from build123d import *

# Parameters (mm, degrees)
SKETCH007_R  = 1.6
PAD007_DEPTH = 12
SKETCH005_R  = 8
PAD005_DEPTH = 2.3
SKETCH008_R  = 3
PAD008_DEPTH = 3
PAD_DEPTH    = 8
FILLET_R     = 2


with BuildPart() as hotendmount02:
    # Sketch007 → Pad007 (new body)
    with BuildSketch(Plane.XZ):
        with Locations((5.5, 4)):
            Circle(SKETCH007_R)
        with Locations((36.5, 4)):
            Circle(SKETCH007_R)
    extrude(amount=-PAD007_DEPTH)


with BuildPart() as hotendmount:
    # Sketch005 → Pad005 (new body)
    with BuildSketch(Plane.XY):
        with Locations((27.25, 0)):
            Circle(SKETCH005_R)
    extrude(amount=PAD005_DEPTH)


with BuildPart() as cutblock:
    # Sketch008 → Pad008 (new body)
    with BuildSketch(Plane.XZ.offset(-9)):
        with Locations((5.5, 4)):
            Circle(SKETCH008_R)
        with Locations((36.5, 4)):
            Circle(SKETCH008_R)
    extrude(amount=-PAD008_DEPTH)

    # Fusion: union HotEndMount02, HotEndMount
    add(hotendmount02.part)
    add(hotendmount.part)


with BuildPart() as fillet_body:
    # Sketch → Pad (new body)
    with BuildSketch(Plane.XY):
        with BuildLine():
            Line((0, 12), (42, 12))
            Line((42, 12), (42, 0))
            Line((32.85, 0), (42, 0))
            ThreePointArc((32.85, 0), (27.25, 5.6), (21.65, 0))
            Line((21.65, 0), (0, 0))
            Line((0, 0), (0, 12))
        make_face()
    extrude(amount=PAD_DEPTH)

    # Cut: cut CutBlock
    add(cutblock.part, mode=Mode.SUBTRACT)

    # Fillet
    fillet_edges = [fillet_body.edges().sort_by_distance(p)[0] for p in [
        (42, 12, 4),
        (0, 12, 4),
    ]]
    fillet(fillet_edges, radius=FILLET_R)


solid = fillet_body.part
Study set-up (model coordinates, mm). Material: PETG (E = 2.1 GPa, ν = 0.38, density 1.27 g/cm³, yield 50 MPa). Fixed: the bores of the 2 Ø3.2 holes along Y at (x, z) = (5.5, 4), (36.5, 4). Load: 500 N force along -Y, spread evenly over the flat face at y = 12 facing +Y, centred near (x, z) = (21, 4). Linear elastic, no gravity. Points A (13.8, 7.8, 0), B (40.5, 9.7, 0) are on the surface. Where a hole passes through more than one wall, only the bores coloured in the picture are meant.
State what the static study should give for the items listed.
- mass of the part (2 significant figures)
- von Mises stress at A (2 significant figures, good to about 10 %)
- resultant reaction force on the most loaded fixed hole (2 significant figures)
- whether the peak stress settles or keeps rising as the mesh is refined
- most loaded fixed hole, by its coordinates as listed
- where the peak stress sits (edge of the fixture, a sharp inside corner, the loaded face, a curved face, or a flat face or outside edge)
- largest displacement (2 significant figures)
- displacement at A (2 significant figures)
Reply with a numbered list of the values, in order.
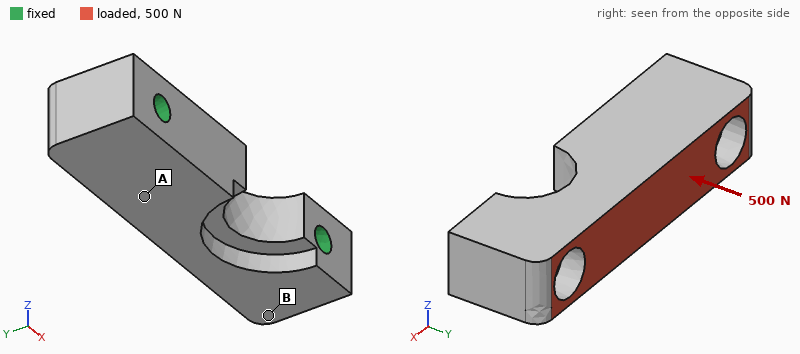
1. 4.1 g
2. 4.2 MPa
3. 290 N
4. keeps rising
5. (5.5, 4)
6. edge of the fixture
7. 83 µm
8. 49 µm
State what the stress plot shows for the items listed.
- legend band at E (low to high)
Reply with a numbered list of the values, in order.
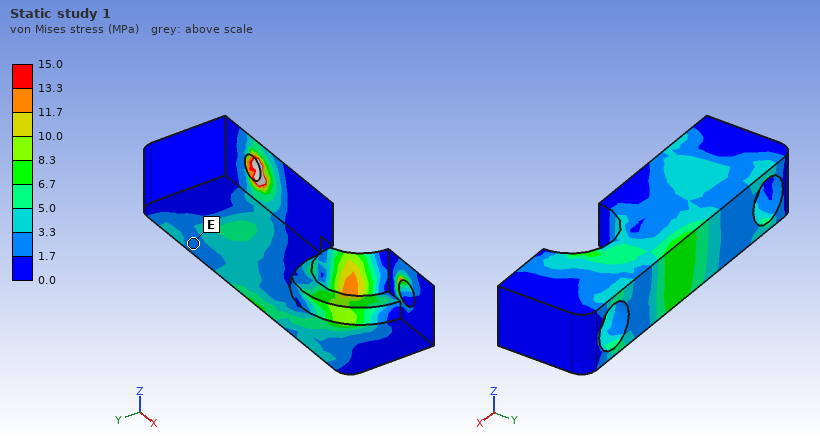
1. 1.7 to 3.3 MPa
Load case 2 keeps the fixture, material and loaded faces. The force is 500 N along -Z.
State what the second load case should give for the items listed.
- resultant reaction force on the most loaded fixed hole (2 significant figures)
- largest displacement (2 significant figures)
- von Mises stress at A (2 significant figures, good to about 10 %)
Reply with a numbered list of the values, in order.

1. 250 N
2. 0.26 mm
3. 8.8 MPa
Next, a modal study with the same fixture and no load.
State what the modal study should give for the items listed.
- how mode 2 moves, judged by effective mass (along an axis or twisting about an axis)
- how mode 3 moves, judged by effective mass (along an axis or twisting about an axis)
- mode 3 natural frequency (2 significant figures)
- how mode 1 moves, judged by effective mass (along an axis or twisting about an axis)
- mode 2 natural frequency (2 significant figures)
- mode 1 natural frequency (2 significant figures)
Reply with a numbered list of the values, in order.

1. along Y
2. twisting about X
3. 9800 Hz
4. along Z
5. 8400 Hz
6. 6500 Hz
